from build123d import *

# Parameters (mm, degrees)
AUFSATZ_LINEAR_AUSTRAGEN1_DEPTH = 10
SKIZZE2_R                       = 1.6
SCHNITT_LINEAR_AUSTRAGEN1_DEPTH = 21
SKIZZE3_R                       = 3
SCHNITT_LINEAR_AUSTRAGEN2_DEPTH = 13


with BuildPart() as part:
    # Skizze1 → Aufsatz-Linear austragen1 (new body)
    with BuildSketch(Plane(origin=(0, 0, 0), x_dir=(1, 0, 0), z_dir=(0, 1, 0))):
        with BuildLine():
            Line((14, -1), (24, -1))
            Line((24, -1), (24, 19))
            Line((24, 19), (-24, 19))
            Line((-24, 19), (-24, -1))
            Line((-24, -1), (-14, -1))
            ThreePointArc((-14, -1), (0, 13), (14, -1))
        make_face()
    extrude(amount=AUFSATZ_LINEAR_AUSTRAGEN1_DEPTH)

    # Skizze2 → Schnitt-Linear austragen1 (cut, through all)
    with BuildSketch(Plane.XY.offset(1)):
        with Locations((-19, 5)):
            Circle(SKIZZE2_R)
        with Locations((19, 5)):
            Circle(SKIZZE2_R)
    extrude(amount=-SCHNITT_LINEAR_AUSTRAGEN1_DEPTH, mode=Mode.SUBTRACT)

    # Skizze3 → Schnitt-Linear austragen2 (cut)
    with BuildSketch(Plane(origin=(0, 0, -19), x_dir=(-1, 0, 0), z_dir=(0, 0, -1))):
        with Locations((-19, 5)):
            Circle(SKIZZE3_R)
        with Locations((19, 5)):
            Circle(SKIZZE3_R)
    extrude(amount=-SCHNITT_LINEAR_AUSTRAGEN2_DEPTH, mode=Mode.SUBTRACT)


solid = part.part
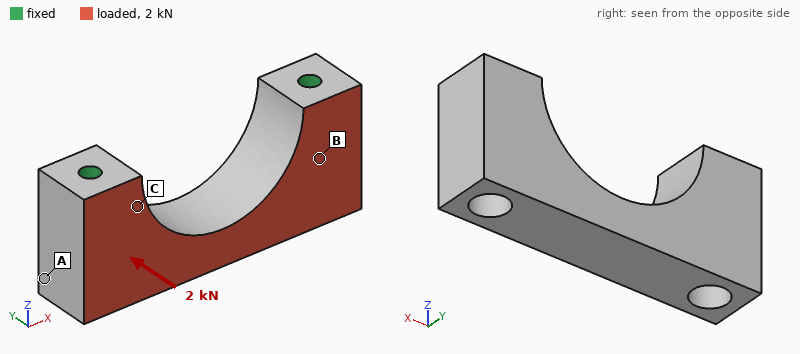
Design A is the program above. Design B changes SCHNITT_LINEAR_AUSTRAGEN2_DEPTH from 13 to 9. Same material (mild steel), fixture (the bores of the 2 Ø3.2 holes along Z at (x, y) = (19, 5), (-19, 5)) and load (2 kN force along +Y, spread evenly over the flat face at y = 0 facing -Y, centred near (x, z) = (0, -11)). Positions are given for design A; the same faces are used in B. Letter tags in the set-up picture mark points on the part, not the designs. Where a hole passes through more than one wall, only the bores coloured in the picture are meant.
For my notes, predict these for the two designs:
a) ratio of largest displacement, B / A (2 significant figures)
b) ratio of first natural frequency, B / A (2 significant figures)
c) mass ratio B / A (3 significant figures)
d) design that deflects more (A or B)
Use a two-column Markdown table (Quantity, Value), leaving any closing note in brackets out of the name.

| Quantity | Value |
|---|---|
| ratio of largest displacement, B / A | 0.48 |
| ratio of first natural frequency, B / A | 1.4 |
| mass ratio B / A | 1.03 |
| design that deflects more | A |
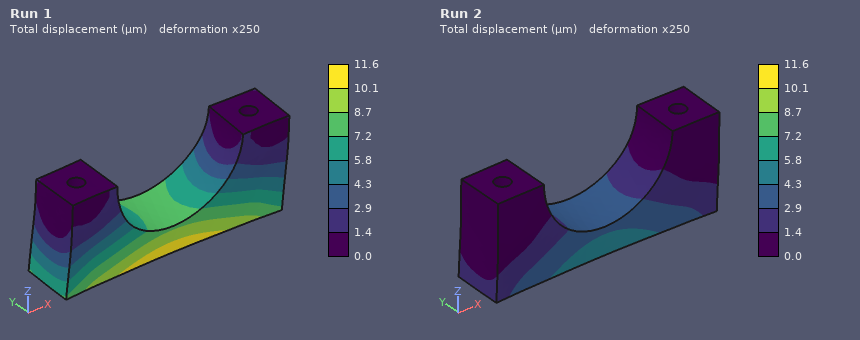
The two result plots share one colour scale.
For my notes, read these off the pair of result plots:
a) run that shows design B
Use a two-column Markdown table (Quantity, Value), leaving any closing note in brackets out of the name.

| Quantity | Value |
|---|---|
| run that shows design B | Run 2 |
